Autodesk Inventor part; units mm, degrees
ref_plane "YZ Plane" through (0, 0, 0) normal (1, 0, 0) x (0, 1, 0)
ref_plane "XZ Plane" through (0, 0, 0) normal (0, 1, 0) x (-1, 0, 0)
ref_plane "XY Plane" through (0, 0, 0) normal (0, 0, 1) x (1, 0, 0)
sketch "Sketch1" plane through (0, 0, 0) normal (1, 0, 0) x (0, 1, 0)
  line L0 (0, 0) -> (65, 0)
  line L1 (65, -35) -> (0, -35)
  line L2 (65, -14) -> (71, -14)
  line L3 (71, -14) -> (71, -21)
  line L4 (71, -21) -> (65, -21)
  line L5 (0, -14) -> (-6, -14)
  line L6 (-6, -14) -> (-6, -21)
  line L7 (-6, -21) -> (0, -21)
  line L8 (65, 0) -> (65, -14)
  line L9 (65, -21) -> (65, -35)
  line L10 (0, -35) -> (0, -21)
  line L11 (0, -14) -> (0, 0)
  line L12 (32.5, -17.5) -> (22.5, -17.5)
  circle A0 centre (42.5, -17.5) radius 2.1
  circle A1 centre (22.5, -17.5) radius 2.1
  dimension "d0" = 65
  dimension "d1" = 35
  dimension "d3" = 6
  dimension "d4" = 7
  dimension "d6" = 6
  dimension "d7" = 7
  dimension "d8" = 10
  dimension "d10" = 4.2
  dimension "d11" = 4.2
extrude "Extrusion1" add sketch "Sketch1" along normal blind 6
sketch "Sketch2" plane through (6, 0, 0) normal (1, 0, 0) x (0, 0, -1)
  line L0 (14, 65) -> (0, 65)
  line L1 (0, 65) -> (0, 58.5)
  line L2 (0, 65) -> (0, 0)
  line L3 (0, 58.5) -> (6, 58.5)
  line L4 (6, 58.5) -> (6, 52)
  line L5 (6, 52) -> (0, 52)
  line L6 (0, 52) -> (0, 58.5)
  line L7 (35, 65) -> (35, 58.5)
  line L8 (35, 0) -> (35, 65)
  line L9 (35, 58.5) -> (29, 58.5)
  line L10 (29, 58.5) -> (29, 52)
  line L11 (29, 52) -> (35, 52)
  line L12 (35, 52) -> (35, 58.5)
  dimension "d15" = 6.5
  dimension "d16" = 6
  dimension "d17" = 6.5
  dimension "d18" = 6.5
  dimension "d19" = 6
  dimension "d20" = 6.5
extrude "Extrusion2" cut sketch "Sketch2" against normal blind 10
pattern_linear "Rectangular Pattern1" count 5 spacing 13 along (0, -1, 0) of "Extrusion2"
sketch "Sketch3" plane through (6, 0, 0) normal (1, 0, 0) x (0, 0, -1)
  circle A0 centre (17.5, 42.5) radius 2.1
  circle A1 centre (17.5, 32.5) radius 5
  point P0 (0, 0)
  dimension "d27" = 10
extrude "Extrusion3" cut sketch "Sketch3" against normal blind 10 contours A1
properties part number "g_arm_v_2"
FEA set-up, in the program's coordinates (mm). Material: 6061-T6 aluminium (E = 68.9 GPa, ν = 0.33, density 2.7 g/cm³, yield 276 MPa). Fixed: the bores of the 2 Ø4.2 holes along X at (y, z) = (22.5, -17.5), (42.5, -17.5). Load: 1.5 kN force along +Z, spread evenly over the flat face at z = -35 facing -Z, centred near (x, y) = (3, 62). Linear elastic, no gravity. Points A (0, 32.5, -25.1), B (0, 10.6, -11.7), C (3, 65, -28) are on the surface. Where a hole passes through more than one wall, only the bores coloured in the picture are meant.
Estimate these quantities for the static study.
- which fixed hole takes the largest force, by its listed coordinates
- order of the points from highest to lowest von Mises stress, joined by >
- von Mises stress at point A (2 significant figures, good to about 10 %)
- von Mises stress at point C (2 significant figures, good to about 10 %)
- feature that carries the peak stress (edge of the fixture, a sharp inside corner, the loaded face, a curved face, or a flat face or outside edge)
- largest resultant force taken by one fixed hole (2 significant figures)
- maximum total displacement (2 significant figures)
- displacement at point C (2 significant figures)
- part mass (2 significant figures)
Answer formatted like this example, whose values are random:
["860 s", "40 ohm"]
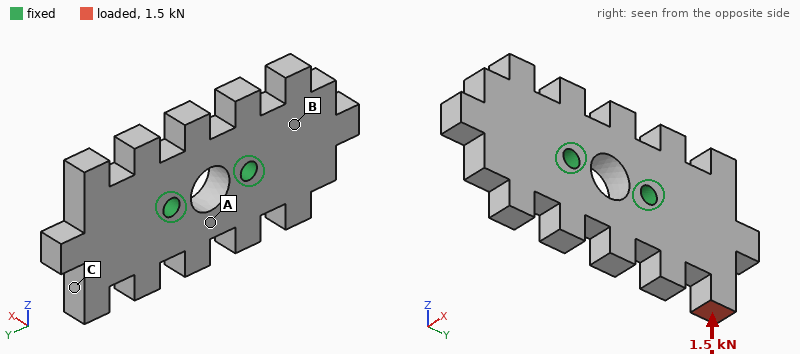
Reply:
["(42.5, -17.5)", "C > A > B", "27 MPa", "45 MPa", "edge of the fixture", "2.3 kN", "59 µm", "47 µm", "30 g"]
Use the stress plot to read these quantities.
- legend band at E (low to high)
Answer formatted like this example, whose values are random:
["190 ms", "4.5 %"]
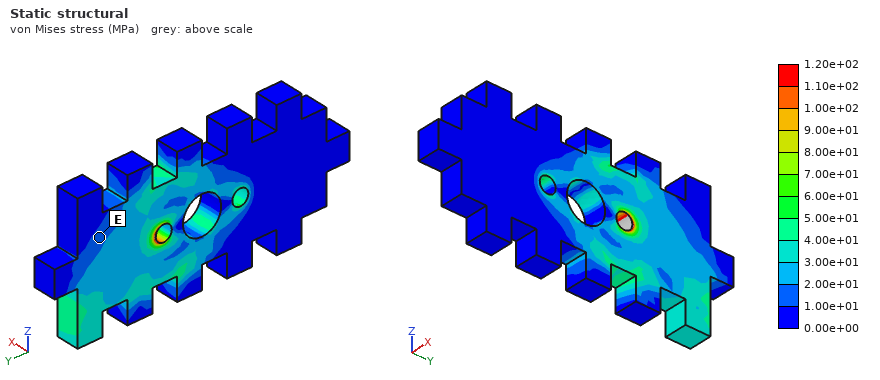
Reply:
["1.00e+01 to 2.00e+01 MPa"]
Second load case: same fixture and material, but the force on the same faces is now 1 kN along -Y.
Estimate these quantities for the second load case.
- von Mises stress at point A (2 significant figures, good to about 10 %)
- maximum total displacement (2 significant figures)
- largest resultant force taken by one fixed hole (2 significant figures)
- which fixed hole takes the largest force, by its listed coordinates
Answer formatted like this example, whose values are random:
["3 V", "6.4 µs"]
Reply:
["20 MPa", "73 µm", "970 N", "(42.5, -17.5)"]
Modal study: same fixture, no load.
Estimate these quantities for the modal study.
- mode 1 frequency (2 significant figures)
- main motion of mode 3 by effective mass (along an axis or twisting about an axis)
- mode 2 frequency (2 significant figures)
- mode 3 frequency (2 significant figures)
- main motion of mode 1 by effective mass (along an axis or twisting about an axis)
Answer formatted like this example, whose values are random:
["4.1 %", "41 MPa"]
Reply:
["6600 Hz", "twisting about Y", "7200 Hz", "9600 Hz", "along X"]
